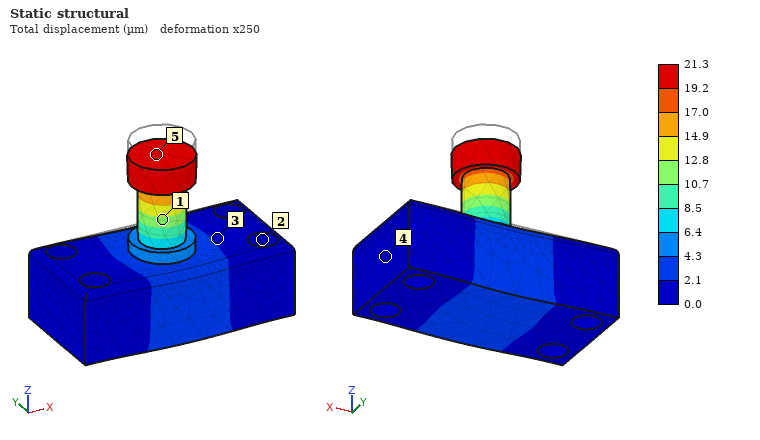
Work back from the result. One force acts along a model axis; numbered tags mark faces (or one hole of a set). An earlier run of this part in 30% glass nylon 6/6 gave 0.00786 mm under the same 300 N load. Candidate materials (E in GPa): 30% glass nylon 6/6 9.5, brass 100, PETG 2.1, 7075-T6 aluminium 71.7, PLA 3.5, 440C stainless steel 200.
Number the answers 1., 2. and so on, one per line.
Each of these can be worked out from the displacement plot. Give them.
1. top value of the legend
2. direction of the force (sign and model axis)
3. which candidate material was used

1. 21.3 µm
2. -Z
3. PLA
